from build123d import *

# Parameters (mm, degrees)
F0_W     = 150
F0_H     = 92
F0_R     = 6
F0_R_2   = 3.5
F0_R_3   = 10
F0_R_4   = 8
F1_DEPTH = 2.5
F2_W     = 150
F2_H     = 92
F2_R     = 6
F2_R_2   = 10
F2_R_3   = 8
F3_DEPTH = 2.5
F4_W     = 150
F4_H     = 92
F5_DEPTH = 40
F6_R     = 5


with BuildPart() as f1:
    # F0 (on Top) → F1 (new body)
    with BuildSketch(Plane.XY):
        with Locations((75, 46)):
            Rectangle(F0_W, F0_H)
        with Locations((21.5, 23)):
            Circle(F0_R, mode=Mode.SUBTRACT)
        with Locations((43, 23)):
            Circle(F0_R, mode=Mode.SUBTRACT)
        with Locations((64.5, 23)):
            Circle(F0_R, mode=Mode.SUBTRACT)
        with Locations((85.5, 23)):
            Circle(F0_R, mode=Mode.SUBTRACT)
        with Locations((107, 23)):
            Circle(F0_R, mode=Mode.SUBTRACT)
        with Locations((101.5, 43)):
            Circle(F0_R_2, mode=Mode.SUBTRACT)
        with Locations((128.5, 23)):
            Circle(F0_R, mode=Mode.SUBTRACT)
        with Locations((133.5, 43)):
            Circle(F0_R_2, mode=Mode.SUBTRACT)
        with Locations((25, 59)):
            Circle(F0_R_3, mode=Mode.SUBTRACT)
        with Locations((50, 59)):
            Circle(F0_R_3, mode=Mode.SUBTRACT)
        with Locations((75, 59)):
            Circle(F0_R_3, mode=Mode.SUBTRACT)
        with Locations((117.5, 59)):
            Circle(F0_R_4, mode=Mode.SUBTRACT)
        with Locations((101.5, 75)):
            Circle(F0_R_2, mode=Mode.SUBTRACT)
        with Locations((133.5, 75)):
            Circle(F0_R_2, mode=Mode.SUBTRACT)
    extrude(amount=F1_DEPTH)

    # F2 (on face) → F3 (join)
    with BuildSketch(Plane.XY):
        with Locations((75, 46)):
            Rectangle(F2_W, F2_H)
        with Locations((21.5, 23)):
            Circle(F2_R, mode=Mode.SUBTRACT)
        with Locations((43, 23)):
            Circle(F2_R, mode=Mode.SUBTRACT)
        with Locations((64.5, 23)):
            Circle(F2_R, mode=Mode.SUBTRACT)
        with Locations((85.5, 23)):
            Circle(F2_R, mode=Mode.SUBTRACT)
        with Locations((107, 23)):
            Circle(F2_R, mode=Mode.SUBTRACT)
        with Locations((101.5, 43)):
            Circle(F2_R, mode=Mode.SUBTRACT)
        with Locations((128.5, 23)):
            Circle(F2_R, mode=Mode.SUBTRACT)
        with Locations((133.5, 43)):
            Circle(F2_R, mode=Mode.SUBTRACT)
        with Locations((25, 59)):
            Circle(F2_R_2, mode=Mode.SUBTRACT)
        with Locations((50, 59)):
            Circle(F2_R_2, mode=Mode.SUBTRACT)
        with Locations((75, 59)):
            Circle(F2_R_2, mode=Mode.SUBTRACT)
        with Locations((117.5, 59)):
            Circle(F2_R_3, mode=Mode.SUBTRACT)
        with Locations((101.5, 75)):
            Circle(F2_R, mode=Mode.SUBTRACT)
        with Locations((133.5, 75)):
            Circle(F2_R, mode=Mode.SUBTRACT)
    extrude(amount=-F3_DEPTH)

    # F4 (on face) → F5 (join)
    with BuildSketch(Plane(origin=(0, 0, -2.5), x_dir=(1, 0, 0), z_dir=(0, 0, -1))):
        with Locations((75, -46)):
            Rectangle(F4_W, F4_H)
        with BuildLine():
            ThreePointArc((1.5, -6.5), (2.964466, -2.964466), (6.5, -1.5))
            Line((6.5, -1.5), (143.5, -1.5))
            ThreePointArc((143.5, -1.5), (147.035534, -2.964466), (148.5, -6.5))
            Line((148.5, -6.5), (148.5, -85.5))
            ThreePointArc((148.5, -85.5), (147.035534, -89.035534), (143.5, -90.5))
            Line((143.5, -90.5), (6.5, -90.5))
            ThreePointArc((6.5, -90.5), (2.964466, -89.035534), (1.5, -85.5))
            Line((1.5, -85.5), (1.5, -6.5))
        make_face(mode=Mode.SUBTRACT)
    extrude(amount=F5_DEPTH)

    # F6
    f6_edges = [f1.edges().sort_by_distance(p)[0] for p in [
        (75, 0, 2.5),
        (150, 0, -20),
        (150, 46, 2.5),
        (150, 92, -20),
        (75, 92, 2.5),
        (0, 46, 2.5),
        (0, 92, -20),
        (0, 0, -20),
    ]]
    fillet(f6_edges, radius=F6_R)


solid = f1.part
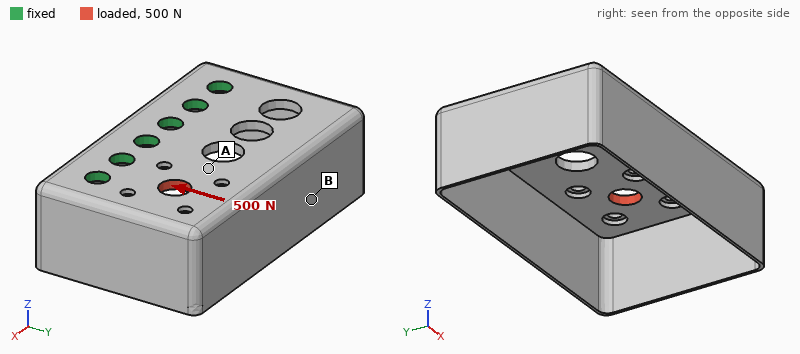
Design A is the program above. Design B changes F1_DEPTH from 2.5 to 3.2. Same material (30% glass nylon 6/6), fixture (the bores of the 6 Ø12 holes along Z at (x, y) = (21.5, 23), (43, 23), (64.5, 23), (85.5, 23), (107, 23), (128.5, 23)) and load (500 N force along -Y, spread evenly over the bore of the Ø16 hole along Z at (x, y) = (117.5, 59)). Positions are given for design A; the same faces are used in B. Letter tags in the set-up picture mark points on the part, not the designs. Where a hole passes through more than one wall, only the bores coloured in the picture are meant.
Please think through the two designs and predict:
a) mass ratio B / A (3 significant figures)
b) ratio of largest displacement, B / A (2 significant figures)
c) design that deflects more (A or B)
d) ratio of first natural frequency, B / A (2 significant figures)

1.10
0.87
A
1.1
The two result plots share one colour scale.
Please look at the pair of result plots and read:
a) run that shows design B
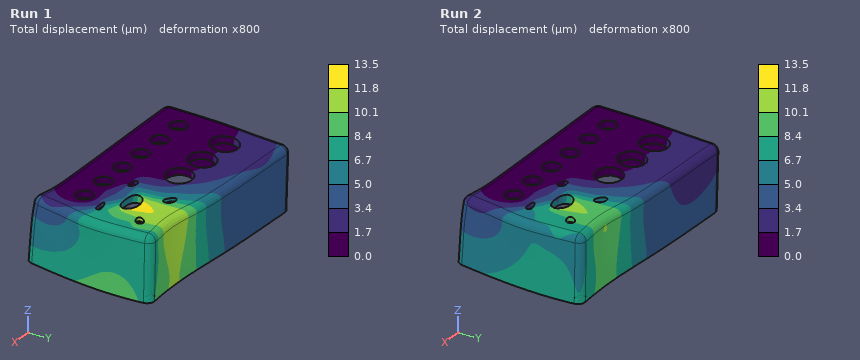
Run 2
